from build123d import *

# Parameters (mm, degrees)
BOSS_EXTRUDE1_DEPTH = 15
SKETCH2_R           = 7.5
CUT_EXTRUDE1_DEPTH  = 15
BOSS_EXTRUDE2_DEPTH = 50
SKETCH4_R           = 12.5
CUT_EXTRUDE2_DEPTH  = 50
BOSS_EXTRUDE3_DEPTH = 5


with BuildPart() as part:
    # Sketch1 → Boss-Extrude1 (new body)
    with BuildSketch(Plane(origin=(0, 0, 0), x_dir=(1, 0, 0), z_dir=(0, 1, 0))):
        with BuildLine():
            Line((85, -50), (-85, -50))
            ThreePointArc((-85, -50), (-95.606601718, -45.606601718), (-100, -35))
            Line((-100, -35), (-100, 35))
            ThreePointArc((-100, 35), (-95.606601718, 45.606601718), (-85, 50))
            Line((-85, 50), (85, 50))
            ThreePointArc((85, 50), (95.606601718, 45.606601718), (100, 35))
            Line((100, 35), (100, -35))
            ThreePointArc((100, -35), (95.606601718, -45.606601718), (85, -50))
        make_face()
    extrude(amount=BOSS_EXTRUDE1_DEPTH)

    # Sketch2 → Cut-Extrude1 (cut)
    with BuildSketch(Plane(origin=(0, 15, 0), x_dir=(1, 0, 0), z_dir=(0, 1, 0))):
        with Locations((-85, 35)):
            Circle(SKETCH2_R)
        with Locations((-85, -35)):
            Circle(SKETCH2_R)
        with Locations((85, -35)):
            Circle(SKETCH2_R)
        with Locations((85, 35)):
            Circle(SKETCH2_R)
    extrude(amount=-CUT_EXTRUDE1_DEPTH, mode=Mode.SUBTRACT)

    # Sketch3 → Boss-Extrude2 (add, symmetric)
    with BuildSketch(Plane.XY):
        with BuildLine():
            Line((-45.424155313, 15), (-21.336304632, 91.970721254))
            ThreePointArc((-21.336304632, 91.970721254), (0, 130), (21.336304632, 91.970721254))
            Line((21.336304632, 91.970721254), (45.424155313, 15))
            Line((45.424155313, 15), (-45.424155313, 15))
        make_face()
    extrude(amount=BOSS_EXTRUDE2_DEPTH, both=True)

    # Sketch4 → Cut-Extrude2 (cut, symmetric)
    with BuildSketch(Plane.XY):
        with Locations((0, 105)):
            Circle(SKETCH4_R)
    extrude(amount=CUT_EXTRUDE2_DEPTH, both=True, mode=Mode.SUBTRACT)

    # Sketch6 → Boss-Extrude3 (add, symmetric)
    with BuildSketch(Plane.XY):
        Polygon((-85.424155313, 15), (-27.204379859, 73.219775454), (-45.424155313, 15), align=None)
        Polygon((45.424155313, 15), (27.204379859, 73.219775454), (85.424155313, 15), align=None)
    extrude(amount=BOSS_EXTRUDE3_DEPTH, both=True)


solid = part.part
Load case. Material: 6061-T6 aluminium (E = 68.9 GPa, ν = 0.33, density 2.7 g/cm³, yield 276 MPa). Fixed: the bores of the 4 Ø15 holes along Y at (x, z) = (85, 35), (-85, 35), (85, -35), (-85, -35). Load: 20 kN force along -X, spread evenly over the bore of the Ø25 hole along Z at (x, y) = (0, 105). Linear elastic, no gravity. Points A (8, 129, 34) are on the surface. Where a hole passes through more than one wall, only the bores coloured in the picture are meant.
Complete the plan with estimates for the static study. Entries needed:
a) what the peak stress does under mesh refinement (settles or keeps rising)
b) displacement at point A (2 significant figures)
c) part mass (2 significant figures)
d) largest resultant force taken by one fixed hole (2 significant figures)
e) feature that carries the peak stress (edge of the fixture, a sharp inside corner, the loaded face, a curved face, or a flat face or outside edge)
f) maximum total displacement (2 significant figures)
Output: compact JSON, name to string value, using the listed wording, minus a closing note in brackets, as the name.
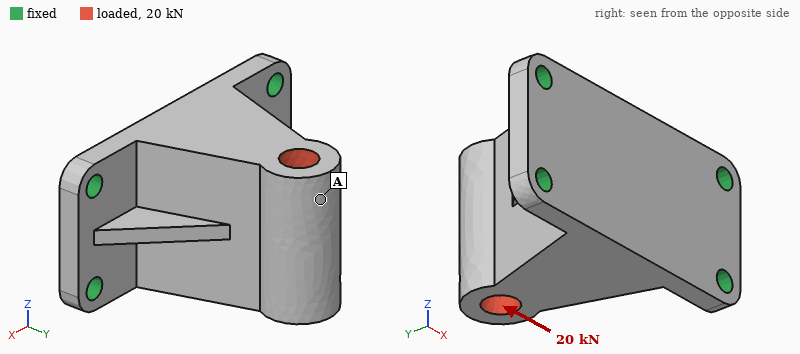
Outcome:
{"what the peak stress does under mesh refinement": "keeps rising", "displacement at point A": "0.14 mm", "part mass": "2.5 kg", "largest resultant force taken by one fixed hole": "8.6 kN", "feature that carries the peak stress": "edge of the fixture", "maximum total displacement": "0.14 mm"}
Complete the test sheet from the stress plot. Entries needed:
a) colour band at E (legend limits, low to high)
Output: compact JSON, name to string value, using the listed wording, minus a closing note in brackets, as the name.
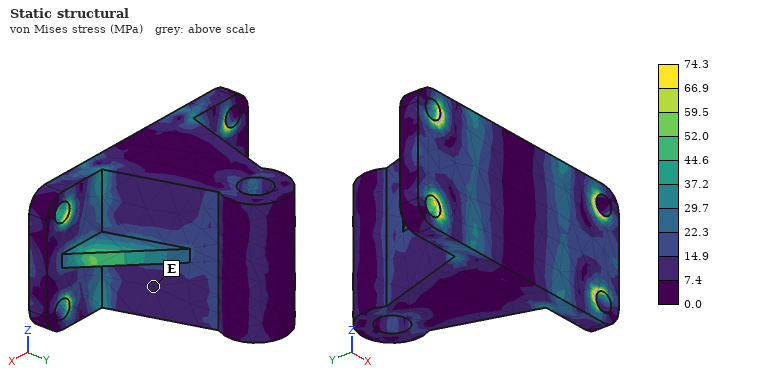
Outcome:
{"colour band at E": "7.4 to 14.9 MPa"}
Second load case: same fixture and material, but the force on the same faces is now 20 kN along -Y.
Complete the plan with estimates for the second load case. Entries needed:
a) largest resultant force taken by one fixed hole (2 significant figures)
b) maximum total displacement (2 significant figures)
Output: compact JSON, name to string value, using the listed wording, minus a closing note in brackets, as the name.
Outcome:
{"largest resultant force taken by one fixed hole": "5.9 kN", "maximum total displacement": "50 µm"}
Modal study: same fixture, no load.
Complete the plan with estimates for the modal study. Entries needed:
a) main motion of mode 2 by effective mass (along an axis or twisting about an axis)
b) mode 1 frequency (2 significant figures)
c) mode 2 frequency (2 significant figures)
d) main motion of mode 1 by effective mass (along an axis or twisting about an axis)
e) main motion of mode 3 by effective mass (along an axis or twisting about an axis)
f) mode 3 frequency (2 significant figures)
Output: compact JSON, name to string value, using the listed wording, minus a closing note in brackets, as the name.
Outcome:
{"main motion of mode 2 by effective mass": "along Y", "mode 1 frequency": "1200 Hz", "mode 2 frequency": "2300 Hz", "main motion of mode 1 by effective mass": "along Z", "main motion of mode 3 by effective mass": "along X", "mode 3 frequency": "2600 Hz"}
